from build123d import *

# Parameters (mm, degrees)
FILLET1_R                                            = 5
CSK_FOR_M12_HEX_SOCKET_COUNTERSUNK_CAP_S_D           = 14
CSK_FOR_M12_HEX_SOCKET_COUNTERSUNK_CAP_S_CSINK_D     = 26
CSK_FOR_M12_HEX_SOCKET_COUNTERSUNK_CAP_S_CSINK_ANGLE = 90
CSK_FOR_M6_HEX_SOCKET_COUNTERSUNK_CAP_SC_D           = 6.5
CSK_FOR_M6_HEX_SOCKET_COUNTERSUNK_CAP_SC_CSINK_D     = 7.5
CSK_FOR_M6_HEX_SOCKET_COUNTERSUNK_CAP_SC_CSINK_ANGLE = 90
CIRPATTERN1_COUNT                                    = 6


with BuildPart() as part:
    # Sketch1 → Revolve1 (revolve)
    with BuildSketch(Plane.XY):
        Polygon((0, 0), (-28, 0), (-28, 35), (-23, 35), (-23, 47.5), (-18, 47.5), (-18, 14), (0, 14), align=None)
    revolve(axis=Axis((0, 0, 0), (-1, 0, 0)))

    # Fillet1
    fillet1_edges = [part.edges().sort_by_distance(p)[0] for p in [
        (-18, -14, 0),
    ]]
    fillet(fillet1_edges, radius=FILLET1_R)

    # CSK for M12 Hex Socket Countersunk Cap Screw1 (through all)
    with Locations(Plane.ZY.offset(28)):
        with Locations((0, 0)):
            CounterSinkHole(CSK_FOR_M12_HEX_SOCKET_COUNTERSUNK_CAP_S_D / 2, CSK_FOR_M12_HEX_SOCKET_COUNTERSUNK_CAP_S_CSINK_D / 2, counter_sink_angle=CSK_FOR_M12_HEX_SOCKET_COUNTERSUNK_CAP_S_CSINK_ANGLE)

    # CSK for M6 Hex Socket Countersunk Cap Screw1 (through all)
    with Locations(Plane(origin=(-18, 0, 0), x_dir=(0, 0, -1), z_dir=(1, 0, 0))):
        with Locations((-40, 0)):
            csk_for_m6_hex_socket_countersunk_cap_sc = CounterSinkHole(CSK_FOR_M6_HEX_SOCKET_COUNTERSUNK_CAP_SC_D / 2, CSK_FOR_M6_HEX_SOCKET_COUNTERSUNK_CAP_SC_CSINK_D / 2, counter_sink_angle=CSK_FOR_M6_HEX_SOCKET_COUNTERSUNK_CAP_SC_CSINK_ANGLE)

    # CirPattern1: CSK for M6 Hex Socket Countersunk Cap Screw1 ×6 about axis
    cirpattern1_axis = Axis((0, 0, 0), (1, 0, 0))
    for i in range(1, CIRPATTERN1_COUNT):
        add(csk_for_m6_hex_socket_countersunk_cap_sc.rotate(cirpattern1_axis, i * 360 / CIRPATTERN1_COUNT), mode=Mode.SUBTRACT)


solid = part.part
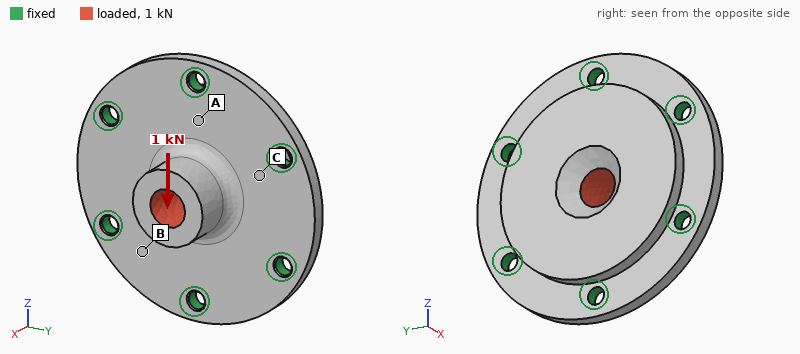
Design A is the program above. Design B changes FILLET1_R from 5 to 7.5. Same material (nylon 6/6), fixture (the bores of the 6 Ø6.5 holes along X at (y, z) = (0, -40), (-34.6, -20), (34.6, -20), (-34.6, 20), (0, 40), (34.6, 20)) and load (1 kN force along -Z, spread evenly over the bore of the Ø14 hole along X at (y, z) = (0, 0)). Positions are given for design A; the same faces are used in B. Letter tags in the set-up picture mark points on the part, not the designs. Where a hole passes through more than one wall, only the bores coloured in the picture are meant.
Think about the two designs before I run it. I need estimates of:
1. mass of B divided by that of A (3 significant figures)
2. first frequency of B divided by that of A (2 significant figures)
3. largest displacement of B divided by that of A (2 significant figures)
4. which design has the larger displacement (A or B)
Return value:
1.01
1.0
0.86
A
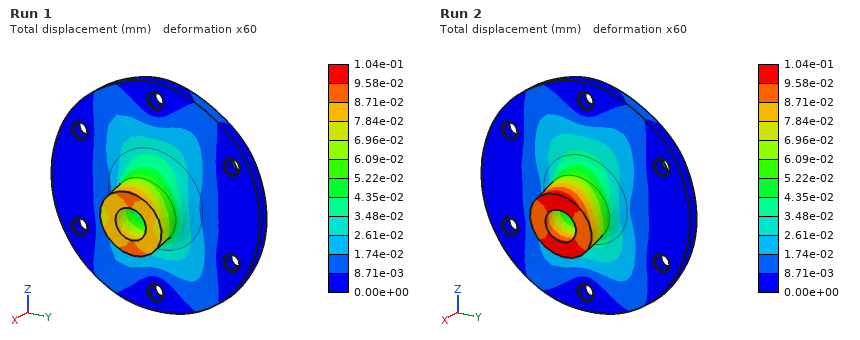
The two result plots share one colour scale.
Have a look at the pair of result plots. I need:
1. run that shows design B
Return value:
Run 1
